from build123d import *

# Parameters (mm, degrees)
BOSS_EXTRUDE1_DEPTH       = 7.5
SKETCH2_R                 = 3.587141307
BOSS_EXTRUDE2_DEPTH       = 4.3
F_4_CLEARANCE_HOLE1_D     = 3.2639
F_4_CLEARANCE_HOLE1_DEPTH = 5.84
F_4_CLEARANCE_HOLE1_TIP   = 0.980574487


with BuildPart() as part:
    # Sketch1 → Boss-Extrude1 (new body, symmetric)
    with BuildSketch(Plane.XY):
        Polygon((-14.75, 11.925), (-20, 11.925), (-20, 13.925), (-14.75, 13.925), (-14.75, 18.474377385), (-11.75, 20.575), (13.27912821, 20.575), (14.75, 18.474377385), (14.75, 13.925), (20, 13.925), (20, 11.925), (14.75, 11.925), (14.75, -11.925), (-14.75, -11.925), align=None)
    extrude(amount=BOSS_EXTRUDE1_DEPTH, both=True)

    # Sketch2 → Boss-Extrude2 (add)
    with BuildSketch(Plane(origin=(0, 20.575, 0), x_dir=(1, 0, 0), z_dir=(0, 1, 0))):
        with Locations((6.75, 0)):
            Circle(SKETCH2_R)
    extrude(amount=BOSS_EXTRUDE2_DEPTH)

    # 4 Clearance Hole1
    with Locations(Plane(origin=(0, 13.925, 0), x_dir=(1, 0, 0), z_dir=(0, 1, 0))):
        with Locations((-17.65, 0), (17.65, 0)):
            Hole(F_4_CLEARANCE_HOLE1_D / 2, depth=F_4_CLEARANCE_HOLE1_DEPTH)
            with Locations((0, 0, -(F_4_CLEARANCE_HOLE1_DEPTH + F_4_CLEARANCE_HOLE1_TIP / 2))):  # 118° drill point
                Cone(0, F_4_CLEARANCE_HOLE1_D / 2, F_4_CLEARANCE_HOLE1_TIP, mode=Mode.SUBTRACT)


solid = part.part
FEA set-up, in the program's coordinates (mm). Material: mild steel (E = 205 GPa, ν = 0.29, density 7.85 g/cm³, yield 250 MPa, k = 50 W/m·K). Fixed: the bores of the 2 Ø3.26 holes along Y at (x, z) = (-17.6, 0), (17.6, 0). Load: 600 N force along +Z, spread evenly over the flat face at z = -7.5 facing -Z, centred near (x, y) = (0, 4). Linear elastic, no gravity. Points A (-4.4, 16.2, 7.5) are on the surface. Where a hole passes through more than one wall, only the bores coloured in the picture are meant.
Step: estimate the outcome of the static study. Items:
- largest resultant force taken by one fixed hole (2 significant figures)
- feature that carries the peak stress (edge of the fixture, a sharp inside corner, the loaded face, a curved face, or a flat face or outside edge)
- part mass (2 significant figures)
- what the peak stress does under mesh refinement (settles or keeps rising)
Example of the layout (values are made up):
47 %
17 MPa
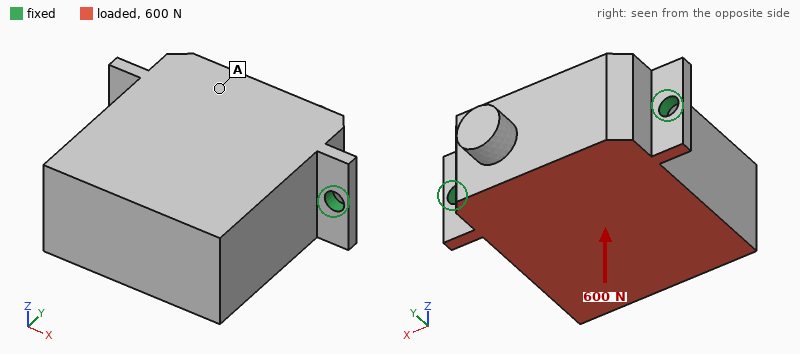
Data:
300 N
edge of the fixture
120 g
keeps rising
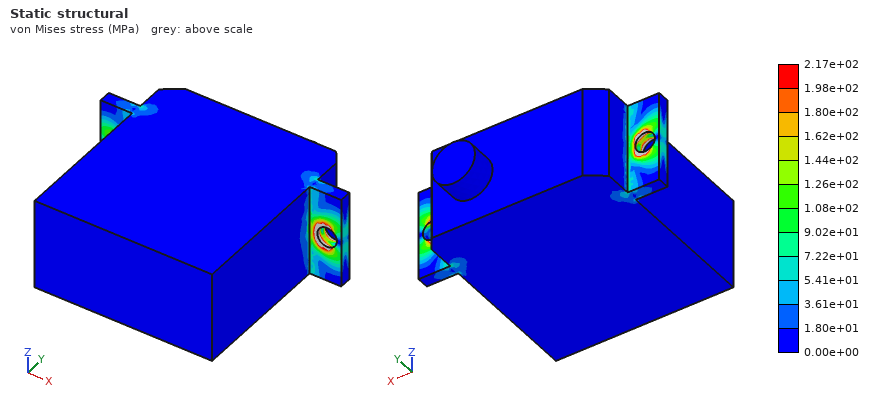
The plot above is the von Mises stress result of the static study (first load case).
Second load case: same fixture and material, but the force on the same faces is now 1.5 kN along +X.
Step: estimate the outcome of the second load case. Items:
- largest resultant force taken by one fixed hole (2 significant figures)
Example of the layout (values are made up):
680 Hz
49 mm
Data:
910 N
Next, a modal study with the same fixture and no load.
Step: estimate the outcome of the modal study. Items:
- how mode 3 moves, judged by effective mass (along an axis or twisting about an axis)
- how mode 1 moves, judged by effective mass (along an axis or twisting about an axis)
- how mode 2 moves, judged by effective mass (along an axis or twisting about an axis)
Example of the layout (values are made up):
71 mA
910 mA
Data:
along Y
along Z
along X
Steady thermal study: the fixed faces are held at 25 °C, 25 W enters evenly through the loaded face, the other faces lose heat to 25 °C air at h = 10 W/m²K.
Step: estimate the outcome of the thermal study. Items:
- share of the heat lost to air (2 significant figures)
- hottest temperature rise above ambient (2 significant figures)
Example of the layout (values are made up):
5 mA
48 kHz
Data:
5.2 %
52 K
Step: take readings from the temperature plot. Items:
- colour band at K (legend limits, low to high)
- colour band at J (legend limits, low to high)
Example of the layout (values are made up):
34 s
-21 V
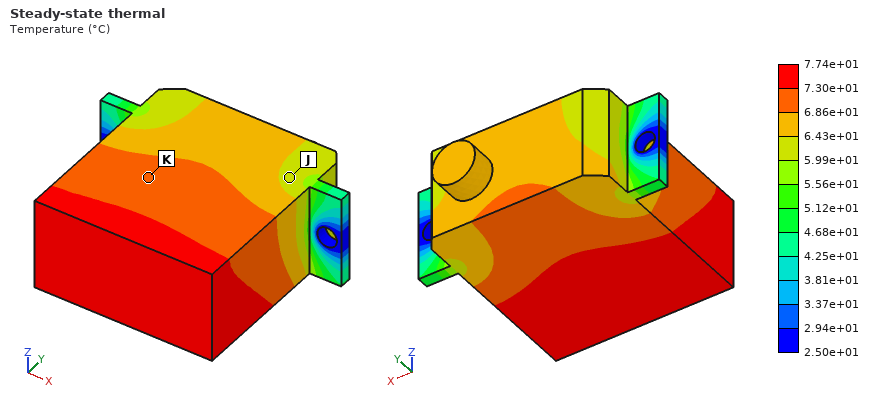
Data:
6.86e+01 to 7.30e+01 °C
5.99e+01 to 6.43e+01 °C
